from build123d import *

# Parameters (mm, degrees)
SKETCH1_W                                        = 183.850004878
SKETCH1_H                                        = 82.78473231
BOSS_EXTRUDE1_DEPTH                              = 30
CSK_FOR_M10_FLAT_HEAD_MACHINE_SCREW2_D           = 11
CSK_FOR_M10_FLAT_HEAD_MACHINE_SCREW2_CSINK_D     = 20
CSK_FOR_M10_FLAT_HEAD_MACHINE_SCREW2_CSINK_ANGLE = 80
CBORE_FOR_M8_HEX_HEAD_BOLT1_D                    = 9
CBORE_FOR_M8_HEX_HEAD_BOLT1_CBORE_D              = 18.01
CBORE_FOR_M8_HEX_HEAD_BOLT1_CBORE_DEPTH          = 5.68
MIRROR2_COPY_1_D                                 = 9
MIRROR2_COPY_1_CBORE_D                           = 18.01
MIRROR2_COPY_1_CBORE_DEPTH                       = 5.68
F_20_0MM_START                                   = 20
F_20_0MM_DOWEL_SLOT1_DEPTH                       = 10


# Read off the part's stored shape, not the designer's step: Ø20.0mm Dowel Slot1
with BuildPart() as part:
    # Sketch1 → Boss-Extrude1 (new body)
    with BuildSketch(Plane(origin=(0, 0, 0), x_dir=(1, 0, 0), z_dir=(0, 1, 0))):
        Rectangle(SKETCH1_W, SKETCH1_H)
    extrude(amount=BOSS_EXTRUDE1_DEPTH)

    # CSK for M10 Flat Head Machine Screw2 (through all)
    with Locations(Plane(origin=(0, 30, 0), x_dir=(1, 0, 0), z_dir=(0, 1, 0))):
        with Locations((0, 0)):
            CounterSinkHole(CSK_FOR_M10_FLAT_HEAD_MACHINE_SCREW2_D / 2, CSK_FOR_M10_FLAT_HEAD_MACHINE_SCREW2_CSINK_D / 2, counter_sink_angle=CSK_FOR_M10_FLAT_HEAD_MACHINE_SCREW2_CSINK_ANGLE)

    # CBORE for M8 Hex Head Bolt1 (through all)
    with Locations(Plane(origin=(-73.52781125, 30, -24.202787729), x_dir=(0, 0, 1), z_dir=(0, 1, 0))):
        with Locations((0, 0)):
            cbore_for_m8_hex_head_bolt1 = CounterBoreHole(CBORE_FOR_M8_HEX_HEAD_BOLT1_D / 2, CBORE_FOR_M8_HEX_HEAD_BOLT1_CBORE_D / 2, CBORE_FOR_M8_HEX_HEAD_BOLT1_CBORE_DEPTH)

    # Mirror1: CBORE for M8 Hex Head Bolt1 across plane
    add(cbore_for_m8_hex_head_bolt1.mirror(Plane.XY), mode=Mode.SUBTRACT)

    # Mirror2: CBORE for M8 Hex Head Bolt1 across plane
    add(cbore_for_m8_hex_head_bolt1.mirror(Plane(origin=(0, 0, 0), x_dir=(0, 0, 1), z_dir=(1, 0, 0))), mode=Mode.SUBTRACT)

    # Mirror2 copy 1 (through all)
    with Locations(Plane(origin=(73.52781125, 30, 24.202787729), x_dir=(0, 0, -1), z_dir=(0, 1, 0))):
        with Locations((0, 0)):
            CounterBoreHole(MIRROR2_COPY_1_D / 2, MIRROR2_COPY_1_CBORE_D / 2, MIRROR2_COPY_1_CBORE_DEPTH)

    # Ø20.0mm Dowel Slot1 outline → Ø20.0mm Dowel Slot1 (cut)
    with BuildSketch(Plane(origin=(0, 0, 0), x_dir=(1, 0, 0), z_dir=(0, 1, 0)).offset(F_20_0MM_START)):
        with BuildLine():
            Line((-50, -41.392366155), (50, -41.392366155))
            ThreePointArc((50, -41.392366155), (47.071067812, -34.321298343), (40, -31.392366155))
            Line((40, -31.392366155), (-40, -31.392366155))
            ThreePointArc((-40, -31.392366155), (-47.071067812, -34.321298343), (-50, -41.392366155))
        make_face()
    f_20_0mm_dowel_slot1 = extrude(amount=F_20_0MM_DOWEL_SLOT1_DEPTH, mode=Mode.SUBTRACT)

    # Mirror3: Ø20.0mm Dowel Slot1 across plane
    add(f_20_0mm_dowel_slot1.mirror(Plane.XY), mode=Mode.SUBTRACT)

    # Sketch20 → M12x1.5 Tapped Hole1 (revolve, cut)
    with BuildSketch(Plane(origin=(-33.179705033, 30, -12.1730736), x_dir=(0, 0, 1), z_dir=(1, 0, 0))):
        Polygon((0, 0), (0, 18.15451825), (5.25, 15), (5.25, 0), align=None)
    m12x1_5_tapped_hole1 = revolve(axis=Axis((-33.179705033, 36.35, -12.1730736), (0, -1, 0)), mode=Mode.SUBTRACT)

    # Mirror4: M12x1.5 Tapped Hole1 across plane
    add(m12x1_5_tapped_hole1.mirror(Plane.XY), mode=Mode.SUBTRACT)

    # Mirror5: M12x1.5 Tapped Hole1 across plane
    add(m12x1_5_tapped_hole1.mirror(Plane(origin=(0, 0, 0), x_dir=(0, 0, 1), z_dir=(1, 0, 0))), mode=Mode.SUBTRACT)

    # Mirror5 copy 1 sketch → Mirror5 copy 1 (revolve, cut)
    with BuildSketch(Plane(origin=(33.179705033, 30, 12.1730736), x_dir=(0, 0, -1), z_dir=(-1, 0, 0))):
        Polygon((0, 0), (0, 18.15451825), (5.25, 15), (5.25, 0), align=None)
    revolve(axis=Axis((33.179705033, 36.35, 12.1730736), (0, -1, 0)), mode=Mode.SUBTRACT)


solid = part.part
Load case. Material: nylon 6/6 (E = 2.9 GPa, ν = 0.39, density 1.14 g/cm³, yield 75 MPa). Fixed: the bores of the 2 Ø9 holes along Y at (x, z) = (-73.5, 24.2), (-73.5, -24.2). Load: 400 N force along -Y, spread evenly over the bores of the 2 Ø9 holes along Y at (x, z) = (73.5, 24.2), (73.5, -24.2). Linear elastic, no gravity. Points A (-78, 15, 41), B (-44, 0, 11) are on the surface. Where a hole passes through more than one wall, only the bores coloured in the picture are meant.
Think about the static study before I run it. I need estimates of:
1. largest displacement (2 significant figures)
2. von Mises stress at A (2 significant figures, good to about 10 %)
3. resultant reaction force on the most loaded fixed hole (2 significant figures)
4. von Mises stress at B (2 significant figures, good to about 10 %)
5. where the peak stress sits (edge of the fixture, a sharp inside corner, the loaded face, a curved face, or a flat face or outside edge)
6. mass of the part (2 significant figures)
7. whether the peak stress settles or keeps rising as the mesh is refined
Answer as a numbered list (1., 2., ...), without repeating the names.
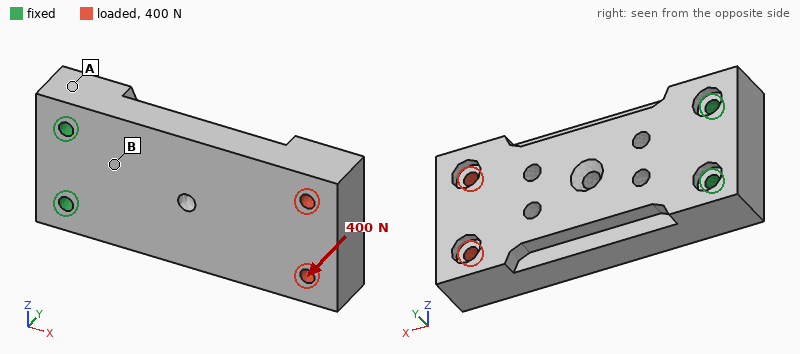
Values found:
1. 1.4 mm
2. 1.9 MPa
3. 200 N
4. 4.0 MPa
5. edge of the fixture
6. 470 g
7. keeps rising
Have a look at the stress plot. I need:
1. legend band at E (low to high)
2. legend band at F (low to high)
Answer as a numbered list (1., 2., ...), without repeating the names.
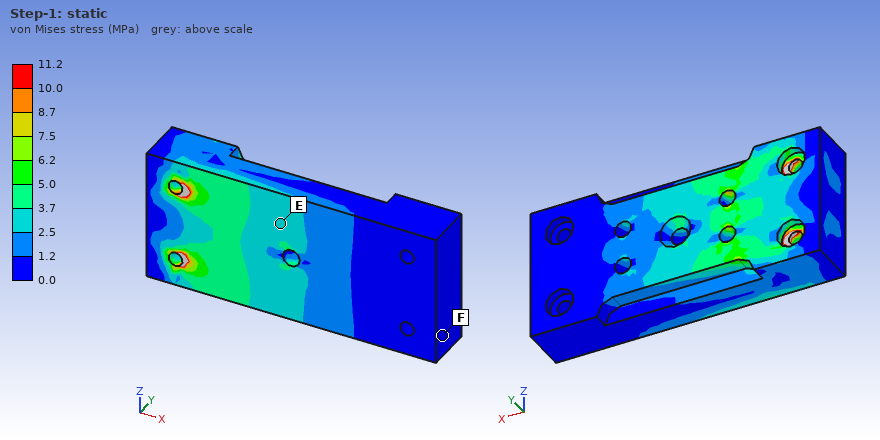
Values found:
1. 2.5 to 3.7 MPa
2. 0.0 to 1.2 MPa
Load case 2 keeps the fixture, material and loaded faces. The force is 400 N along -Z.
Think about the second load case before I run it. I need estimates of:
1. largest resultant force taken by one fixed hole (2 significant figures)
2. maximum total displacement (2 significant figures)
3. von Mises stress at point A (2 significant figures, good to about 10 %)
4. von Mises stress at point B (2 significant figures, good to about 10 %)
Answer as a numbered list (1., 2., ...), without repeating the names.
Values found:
1. 1.1 kN
2. 0.21 mm
3. 0.63 MPa
4. 0.79 MPa
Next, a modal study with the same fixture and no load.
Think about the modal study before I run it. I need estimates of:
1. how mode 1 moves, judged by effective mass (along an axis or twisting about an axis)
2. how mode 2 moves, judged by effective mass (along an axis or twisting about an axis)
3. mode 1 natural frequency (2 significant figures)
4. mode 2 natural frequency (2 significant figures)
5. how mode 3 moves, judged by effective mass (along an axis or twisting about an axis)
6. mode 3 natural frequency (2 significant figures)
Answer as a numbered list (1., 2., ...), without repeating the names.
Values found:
1. along Y
2. along Z
3. 240 Hz
4. 590 Hz
5. twisting about X
6. 880 Hz
